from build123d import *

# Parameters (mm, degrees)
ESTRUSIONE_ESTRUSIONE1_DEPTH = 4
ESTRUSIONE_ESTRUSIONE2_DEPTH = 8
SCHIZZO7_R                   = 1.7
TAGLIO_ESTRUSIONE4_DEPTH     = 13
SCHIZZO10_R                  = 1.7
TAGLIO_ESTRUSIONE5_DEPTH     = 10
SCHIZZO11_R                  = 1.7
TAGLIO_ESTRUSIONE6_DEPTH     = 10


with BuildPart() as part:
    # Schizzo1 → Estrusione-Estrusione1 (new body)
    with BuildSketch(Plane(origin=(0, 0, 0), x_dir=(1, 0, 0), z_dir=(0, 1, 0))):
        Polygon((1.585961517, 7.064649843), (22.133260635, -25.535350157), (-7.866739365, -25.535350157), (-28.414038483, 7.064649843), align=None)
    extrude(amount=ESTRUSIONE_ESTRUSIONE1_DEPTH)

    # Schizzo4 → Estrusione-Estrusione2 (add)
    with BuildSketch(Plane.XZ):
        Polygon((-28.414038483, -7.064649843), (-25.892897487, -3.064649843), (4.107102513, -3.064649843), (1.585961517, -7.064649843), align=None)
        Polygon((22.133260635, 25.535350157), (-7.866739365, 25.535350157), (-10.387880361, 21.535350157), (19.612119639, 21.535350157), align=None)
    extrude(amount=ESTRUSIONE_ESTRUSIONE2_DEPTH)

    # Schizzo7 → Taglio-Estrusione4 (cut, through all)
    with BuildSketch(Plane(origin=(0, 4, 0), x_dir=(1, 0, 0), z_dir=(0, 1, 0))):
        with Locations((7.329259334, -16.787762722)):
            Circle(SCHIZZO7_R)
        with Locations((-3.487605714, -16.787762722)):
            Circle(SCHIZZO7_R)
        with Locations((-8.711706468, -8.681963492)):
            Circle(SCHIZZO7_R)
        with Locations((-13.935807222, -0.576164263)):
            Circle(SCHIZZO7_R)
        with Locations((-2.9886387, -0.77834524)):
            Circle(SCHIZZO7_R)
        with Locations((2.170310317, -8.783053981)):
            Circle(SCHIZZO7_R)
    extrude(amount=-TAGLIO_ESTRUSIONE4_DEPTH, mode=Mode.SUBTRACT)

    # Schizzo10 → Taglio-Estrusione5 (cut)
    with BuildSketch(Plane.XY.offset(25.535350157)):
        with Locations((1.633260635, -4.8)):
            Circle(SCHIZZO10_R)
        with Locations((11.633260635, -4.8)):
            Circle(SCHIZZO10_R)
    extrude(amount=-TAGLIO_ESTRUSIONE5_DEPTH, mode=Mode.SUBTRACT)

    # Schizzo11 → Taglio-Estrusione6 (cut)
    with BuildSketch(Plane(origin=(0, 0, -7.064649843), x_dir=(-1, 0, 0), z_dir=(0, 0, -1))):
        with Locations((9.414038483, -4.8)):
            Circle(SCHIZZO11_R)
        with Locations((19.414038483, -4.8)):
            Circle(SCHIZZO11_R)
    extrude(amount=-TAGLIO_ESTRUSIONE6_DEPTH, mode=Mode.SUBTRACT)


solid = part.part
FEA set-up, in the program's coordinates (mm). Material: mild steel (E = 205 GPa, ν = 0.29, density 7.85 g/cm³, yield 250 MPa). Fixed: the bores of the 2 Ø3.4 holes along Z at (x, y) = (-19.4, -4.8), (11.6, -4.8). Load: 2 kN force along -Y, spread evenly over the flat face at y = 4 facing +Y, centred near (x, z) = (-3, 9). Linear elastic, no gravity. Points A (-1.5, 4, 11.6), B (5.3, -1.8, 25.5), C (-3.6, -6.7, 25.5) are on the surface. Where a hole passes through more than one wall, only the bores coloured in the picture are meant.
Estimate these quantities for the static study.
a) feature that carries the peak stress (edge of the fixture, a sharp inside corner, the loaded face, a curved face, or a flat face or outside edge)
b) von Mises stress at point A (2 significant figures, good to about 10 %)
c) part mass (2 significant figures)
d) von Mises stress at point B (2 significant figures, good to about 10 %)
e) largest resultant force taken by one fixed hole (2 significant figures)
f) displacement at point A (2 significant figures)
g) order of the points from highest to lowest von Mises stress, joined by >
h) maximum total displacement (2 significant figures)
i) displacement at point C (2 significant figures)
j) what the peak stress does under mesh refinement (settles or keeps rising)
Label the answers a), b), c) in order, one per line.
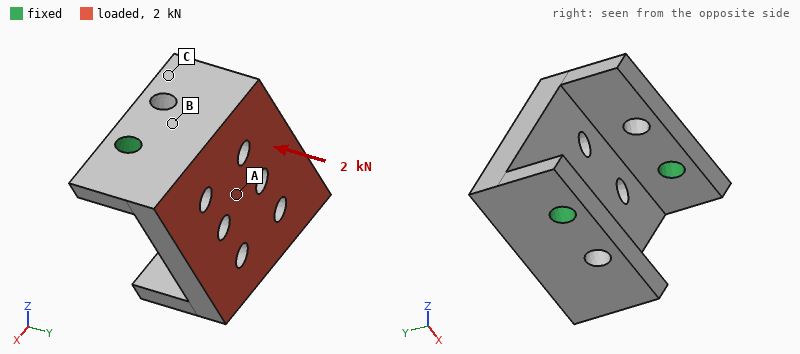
a) edge of the fixture
b) 55 MPa
c) 43 g
d) 24 MPa
e) 1.4 kN
f) 14 µm
g) A > B > C
h) 17 µm
i) 7.5 µm
j) keeps rising
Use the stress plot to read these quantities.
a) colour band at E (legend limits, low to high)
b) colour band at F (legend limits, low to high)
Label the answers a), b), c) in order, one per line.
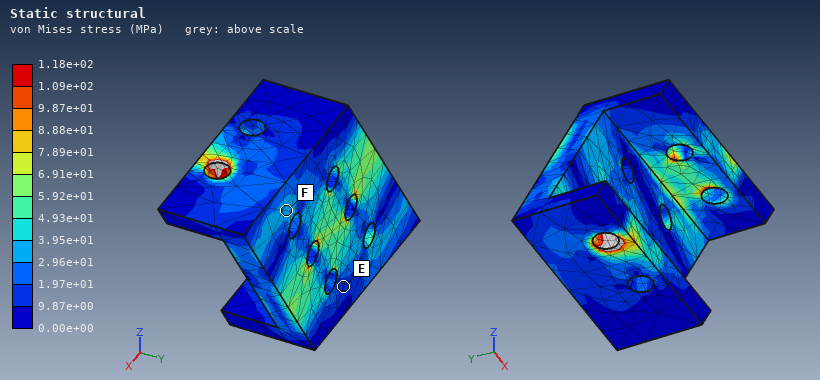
a) 9.87e+00 to 1.97e+01 MPa
b) 2.96e+01 to 3.95e+01 MPa
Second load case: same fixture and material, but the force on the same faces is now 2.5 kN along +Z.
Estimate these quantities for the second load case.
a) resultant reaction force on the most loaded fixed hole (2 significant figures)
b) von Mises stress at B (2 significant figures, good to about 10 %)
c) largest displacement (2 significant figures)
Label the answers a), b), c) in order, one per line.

a) 1.3 kN
b) 30 MPa
c) 21 µm
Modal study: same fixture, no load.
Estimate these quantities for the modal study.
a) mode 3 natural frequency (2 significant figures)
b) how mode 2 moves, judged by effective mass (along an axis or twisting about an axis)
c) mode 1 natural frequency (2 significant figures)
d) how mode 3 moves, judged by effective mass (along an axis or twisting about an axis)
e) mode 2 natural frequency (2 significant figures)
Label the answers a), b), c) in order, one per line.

a) 14 kHz
b) along Y
c) 8800 Hz
d) along Z
e) 11 kHz
